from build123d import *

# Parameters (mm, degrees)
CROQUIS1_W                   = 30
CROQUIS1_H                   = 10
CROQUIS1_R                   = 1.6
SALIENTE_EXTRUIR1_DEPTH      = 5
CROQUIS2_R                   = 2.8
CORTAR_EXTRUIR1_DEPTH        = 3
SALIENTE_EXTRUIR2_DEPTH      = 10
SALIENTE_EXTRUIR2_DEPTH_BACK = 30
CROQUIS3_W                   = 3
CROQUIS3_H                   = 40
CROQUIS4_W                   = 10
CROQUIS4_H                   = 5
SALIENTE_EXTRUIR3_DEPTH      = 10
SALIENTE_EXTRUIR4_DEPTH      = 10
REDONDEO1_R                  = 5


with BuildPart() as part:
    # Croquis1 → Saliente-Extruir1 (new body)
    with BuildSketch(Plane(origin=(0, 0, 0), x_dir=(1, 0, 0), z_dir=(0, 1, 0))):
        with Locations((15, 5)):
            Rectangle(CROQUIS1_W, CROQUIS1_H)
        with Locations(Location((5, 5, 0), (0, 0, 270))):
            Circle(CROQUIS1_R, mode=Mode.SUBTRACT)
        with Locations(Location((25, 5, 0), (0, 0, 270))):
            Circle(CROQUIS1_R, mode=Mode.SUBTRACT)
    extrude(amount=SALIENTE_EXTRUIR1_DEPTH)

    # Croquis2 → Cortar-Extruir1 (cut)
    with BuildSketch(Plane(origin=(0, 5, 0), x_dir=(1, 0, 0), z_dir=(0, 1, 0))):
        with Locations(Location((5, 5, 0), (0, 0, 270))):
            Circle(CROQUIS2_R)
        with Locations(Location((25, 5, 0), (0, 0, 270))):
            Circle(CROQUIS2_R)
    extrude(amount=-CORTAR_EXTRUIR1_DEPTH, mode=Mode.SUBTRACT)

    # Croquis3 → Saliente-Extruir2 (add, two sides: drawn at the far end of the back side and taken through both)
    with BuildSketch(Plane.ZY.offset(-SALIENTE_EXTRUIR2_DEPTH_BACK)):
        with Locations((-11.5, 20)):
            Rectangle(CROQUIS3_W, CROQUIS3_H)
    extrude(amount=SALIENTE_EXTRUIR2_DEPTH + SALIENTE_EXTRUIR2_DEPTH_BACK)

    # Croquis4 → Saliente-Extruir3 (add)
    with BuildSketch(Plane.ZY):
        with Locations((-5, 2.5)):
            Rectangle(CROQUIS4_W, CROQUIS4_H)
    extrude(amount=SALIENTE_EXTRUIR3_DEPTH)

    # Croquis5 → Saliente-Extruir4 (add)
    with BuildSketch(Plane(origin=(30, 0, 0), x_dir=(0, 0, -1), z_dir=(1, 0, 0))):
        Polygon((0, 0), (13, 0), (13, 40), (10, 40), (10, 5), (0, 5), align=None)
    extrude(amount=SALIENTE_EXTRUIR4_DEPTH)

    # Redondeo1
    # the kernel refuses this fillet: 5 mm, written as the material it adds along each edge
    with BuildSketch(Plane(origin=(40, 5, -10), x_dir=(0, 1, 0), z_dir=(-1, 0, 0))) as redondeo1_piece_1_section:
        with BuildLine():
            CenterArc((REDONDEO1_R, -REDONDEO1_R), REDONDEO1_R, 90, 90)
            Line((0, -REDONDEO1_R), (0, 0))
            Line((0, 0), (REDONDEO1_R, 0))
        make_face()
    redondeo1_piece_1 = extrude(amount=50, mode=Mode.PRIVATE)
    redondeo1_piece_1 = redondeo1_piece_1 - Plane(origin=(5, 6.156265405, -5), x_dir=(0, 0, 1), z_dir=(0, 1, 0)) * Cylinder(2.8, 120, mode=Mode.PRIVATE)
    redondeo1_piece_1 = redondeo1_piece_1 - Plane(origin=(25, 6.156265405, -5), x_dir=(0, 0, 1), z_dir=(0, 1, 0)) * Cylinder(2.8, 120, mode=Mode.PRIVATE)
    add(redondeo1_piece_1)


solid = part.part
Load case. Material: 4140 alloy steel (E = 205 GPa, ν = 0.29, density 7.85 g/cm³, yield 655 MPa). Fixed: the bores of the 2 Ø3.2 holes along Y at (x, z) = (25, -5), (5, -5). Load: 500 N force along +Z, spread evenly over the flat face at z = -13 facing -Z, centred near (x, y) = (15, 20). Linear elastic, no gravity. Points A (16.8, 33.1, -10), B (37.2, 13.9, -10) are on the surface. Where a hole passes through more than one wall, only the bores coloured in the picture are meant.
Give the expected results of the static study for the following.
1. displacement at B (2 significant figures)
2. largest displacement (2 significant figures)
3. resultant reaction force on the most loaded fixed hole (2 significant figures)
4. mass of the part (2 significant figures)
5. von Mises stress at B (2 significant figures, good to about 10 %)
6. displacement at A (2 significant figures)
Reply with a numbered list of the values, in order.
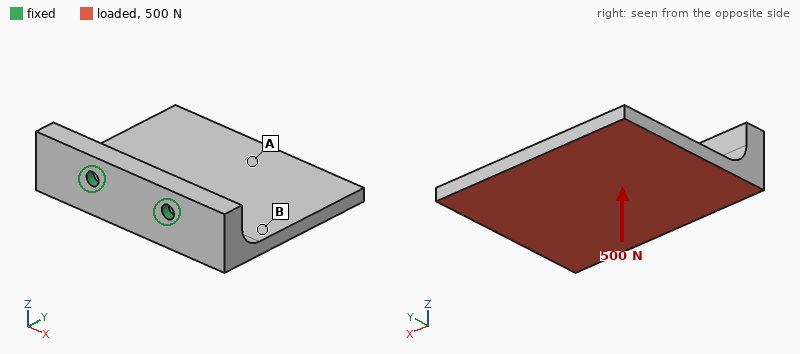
1. 0.035 mm
2. 0.17 mm
3. 250 N
4. 67 g
5. 53 MPa
6. 0.13 mm
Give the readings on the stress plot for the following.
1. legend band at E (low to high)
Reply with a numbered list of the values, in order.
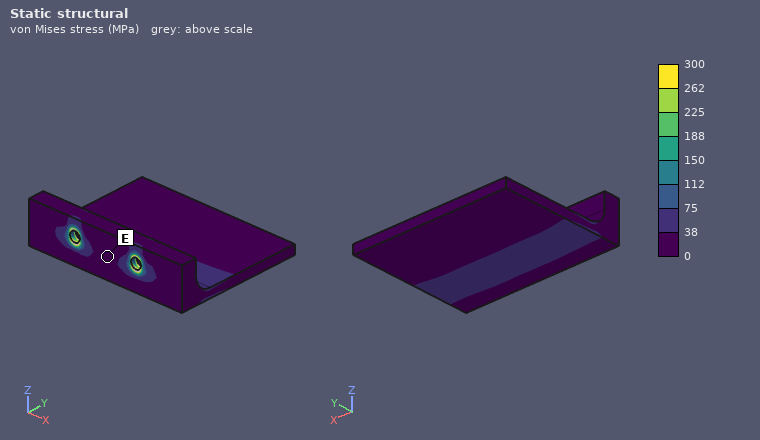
1. 0 to 38 MPa
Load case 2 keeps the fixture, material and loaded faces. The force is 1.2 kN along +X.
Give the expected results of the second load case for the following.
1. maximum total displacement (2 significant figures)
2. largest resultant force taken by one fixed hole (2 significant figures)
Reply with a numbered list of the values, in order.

1. 26 µm
2. 1.3 kN
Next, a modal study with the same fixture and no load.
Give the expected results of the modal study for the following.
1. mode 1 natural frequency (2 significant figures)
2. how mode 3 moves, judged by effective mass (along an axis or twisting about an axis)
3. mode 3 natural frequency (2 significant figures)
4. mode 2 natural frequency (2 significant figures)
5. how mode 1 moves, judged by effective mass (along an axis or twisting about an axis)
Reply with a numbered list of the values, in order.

1. 1600 Hz
2. along X
3. 5600 Hz
4. 3400 Hz
5. along Z
